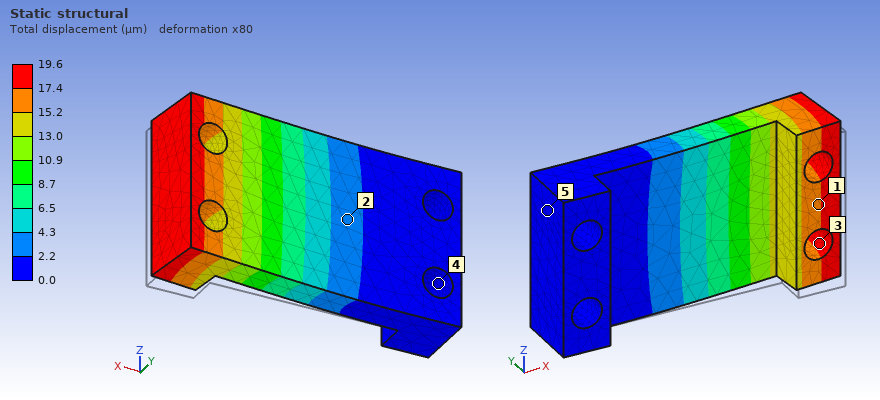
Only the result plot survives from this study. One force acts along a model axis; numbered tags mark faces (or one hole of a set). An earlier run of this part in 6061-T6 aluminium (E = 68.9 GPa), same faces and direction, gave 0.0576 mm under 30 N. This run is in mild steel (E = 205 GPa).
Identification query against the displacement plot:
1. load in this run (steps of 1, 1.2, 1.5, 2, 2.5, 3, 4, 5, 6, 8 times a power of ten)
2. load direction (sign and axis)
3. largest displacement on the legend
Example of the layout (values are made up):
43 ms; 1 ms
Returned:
30 N; +Y; 19.6 µm
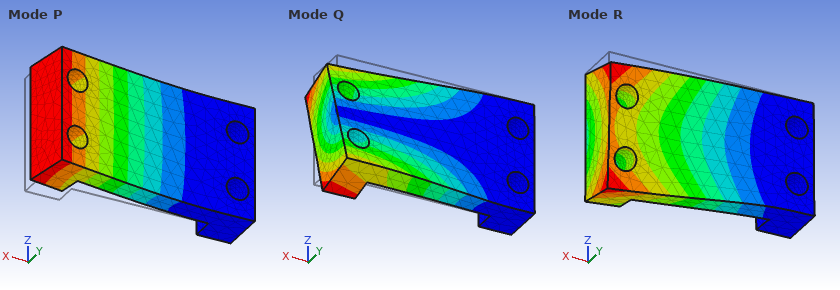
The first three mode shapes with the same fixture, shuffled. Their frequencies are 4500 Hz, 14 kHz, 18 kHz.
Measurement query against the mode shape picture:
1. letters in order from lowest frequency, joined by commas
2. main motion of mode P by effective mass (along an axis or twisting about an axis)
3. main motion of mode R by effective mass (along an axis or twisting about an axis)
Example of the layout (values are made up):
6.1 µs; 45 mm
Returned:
P, Q, R; along Y; along Z
